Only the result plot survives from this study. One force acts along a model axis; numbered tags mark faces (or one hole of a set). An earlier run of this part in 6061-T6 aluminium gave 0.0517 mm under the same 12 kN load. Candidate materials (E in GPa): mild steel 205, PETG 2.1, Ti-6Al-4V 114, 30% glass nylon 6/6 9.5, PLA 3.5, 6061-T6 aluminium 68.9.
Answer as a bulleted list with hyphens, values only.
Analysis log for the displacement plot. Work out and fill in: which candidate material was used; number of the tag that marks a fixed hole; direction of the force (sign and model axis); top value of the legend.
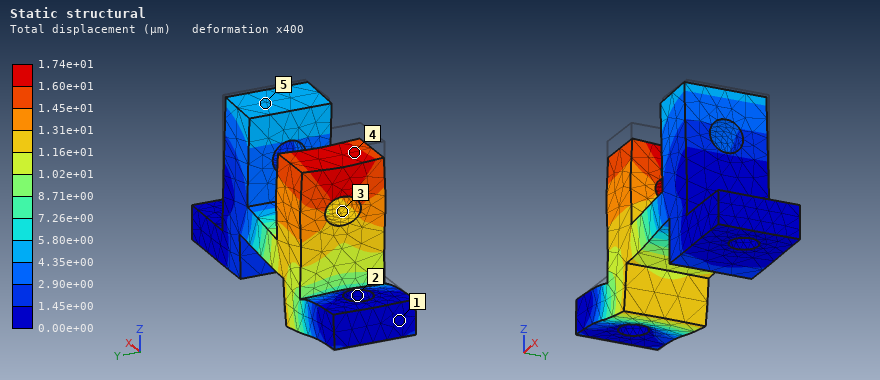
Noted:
- mild steel
- 2
- -Z
- 1.74e+01 µm
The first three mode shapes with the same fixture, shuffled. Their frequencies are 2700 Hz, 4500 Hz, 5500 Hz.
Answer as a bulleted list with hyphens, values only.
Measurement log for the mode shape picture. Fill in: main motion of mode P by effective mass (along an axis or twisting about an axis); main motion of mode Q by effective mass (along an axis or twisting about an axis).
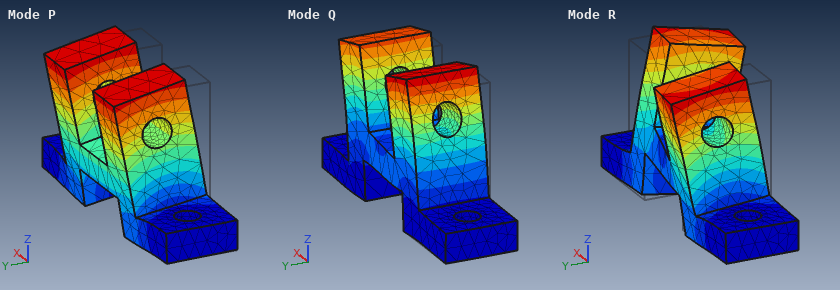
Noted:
- along Y
- along X
